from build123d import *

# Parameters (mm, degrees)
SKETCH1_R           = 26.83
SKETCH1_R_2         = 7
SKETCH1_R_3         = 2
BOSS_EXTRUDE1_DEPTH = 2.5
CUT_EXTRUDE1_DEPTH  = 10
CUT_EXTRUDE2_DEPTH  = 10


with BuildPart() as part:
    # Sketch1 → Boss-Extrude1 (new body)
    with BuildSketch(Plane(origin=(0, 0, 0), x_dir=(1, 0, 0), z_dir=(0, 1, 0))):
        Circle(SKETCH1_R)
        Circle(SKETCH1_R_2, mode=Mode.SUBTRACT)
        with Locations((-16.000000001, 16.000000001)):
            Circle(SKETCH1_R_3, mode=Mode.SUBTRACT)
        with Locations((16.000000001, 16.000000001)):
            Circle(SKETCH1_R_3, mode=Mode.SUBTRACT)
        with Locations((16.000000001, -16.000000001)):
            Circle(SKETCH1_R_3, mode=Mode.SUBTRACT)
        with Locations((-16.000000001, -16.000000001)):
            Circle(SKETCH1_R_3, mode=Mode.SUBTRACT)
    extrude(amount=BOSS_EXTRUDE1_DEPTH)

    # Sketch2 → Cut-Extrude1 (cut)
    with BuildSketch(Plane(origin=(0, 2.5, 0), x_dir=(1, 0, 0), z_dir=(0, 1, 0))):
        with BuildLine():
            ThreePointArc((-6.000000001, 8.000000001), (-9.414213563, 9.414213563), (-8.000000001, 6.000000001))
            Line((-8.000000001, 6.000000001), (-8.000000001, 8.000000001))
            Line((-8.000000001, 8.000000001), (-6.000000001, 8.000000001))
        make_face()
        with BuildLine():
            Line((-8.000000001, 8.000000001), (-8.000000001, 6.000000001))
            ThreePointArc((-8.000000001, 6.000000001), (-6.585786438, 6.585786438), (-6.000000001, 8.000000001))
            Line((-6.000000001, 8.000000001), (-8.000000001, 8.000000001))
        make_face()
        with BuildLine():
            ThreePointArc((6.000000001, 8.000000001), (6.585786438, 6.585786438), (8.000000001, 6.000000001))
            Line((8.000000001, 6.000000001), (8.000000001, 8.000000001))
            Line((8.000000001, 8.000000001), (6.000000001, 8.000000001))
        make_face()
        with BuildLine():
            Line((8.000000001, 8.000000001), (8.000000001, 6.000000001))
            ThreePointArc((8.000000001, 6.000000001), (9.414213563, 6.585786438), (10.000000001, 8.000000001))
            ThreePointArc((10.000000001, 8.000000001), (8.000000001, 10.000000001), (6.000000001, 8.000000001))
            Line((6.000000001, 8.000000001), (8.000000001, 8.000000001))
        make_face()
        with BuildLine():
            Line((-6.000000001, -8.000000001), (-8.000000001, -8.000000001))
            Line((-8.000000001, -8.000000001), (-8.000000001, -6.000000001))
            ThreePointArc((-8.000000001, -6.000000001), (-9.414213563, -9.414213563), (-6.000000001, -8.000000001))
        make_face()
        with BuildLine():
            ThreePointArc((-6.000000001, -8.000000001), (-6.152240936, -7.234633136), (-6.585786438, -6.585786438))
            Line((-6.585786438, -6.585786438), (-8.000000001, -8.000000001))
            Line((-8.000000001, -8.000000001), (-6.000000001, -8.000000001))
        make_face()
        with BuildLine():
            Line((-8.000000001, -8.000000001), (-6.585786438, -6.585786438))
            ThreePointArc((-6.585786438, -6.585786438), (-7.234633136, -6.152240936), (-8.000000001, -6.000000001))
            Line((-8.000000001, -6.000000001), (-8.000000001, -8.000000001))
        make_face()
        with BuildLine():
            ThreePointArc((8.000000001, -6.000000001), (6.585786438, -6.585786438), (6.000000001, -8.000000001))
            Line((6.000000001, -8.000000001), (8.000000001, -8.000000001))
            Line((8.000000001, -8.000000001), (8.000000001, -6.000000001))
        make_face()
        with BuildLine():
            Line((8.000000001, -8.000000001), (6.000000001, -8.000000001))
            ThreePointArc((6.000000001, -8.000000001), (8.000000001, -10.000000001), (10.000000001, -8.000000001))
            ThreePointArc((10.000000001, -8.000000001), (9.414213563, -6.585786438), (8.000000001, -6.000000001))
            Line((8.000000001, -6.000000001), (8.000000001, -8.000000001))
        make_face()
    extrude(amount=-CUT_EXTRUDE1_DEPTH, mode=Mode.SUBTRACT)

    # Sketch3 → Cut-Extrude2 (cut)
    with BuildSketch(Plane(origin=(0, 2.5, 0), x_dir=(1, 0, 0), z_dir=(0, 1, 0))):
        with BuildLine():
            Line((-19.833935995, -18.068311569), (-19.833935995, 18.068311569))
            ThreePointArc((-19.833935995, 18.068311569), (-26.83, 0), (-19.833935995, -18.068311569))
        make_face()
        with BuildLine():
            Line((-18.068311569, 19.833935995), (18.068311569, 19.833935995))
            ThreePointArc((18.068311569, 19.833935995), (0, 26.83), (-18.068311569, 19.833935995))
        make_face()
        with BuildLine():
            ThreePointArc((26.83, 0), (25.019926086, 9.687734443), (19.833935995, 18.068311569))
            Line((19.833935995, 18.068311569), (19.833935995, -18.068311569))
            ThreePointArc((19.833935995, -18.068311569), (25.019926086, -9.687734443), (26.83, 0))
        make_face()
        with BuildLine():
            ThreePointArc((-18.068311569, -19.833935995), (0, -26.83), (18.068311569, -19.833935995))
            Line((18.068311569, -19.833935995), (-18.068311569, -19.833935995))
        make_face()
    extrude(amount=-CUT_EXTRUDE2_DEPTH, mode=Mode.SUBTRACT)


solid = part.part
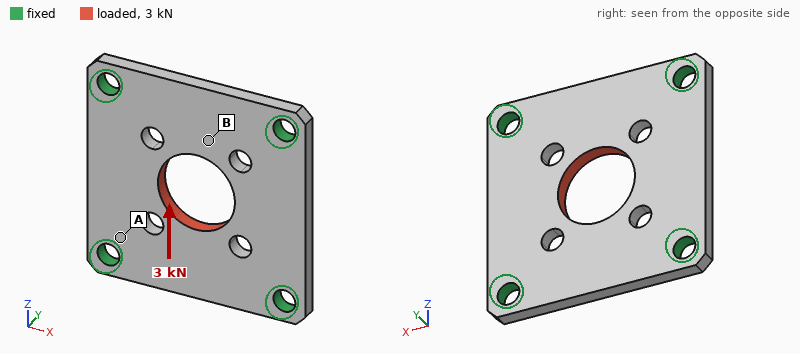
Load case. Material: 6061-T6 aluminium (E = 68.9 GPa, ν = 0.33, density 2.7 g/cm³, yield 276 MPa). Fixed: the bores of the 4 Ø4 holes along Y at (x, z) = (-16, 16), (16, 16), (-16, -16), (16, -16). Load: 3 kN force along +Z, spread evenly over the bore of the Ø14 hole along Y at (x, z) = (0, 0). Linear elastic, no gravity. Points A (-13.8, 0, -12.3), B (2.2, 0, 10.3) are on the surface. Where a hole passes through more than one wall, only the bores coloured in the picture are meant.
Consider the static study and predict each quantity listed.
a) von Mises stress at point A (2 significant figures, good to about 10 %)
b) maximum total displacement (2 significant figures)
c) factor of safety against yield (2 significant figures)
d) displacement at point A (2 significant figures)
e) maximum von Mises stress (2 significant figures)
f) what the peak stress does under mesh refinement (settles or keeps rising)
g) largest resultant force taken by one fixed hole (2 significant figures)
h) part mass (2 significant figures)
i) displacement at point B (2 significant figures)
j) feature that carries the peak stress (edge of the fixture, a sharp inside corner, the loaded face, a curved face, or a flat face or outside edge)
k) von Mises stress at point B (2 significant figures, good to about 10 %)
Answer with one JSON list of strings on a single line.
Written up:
["41 MPa", "12 µm", "3.1", "1.8 µm", "90 MPa", "settles", "830 N", "8.9 g", "11 µm", "a curved face", "18 MPa"]
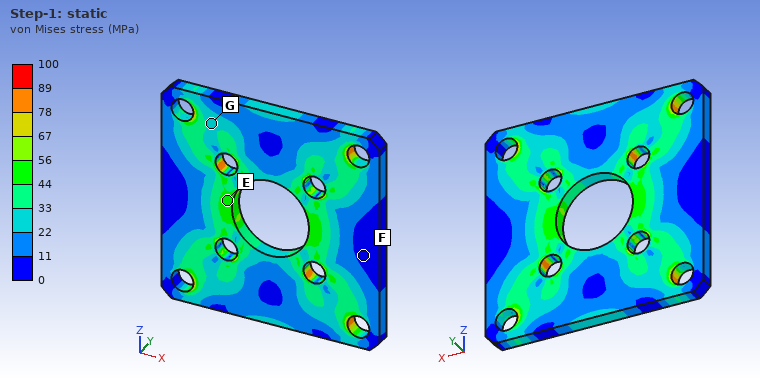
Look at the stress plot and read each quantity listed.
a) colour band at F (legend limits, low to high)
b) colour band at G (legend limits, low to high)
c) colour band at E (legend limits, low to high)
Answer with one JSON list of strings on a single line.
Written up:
["0 to 11 MPa", "22 to 33 MPa", "44 to 56 MPa"]
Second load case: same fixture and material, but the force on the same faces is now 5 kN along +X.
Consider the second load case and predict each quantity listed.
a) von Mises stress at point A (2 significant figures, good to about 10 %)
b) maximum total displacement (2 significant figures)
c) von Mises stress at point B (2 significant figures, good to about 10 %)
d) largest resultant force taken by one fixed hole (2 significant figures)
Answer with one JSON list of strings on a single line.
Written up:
["59 MPa", "20 µm", "60 MPa", "1.4 kN"]
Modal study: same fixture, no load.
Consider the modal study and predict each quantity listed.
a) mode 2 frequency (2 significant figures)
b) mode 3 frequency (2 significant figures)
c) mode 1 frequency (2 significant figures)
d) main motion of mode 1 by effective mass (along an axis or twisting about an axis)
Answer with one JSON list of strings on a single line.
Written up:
["15 kHz", "15 kHz", "11 kHz", "along Y"]
